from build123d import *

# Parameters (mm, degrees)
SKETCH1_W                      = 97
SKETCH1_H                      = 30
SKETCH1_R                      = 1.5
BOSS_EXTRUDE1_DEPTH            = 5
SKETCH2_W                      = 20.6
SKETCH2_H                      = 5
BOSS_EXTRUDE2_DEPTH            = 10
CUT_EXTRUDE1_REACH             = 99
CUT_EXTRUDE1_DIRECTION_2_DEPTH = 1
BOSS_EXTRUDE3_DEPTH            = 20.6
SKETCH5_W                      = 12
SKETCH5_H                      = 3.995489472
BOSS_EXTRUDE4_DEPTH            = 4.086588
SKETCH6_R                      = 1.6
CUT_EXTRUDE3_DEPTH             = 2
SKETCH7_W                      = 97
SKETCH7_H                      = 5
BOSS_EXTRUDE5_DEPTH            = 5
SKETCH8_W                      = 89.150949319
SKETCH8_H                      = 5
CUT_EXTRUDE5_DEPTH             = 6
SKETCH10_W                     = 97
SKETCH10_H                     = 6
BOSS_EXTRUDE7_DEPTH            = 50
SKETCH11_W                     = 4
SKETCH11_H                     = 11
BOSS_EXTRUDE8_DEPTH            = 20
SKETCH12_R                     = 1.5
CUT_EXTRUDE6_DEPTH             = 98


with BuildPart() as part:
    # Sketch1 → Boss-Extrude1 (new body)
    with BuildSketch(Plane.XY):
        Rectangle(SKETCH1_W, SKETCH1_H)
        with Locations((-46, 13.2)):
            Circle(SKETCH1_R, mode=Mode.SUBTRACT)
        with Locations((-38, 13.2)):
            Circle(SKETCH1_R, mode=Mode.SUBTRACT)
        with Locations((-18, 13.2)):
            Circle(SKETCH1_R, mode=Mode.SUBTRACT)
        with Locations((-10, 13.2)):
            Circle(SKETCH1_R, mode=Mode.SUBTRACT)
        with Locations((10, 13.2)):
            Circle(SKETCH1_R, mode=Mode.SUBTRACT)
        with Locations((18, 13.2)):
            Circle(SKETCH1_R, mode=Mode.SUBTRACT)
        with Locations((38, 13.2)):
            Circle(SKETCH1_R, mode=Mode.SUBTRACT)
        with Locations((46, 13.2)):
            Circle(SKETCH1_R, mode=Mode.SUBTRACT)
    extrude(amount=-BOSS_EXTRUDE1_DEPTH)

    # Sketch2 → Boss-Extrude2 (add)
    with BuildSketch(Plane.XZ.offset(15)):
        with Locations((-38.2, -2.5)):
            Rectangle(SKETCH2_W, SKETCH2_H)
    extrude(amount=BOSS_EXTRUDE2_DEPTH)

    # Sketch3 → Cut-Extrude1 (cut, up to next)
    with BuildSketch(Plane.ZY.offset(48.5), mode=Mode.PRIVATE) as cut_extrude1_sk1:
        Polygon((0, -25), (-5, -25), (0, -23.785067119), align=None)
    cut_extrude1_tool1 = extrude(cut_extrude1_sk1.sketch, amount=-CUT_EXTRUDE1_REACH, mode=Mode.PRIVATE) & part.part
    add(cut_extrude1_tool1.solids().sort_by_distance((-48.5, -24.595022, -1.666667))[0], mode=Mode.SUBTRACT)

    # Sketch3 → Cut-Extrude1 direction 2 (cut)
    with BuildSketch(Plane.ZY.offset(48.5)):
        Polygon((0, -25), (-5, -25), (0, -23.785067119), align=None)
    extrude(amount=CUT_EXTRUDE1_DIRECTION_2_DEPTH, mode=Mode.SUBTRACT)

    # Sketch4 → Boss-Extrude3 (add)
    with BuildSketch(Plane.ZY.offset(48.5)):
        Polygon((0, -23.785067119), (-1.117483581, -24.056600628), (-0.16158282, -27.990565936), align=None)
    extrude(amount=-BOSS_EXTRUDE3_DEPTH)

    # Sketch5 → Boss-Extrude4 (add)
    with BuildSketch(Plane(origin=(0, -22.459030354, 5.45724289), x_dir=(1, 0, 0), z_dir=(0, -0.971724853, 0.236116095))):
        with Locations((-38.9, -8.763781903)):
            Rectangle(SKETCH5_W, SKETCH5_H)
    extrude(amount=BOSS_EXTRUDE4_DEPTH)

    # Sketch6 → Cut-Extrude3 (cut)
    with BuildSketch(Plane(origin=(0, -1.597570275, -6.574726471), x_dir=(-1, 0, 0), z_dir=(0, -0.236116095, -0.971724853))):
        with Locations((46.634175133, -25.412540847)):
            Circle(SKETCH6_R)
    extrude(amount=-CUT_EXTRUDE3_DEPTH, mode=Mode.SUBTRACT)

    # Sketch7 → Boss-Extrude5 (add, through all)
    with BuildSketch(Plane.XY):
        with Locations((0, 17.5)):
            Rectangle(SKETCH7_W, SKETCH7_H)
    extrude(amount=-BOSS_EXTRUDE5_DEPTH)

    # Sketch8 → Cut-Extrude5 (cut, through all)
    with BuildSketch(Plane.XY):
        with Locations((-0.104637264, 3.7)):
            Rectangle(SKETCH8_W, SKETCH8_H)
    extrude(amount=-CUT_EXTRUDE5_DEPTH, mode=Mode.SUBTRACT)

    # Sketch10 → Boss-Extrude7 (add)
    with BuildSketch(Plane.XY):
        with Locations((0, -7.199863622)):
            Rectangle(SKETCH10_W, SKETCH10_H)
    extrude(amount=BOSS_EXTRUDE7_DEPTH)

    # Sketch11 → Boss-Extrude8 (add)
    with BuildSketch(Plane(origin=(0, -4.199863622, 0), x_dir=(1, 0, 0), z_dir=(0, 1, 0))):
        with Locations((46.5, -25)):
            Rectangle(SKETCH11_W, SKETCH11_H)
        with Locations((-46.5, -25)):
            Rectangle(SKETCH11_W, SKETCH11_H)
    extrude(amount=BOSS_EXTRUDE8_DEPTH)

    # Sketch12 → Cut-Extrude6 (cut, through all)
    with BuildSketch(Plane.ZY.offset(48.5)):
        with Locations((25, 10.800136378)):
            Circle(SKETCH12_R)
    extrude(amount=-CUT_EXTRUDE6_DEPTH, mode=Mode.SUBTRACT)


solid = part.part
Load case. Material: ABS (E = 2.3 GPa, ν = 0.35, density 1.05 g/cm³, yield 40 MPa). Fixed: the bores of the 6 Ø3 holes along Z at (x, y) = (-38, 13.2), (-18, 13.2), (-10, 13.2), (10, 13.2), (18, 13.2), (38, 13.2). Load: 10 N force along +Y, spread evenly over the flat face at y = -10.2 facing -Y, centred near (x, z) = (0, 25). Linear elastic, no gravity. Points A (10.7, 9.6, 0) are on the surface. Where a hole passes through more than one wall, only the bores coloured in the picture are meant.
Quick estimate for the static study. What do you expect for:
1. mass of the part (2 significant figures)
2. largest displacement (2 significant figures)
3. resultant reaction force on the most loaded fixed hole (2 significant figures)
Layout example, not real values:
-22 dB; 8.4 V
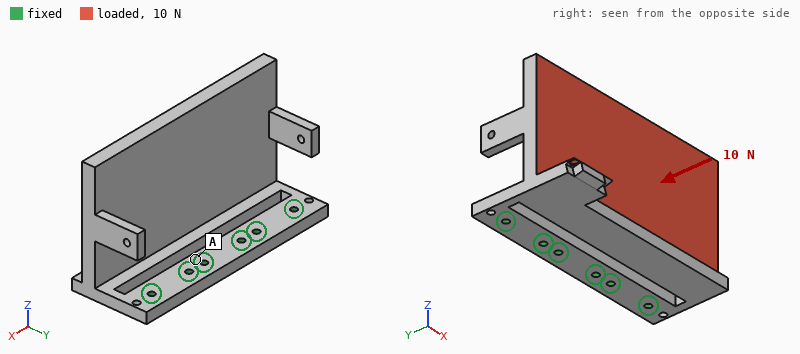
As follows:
49 g; 1.3 mm; 6.7 N
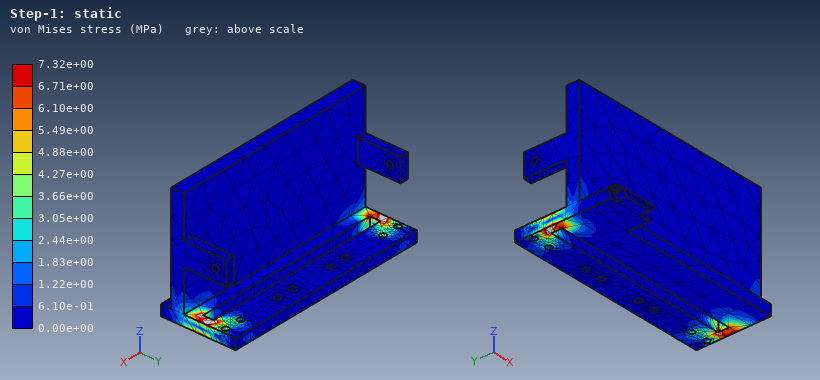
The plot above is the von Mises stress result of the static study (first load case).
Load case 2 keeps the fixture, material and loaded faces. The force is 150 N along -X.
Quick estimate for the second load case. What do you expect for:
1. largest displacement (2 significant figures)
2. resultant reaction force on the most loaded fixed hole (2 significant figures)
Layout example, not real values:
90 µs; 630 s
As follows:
0.70 mm; 96 N
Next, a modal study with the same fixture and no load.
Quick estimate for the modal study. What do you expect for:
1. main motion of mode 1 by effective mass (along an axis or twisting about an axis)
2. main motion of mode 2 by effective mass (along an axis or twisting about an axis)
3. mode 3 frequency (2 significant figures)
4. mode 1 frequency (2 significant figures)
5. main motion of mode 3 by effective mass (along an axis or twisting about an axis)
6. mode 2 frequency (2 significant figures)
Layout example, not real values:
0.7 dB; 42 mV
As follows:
along Y; along X; 440 Hz; 90 Hz; along Z; 390 Hz
